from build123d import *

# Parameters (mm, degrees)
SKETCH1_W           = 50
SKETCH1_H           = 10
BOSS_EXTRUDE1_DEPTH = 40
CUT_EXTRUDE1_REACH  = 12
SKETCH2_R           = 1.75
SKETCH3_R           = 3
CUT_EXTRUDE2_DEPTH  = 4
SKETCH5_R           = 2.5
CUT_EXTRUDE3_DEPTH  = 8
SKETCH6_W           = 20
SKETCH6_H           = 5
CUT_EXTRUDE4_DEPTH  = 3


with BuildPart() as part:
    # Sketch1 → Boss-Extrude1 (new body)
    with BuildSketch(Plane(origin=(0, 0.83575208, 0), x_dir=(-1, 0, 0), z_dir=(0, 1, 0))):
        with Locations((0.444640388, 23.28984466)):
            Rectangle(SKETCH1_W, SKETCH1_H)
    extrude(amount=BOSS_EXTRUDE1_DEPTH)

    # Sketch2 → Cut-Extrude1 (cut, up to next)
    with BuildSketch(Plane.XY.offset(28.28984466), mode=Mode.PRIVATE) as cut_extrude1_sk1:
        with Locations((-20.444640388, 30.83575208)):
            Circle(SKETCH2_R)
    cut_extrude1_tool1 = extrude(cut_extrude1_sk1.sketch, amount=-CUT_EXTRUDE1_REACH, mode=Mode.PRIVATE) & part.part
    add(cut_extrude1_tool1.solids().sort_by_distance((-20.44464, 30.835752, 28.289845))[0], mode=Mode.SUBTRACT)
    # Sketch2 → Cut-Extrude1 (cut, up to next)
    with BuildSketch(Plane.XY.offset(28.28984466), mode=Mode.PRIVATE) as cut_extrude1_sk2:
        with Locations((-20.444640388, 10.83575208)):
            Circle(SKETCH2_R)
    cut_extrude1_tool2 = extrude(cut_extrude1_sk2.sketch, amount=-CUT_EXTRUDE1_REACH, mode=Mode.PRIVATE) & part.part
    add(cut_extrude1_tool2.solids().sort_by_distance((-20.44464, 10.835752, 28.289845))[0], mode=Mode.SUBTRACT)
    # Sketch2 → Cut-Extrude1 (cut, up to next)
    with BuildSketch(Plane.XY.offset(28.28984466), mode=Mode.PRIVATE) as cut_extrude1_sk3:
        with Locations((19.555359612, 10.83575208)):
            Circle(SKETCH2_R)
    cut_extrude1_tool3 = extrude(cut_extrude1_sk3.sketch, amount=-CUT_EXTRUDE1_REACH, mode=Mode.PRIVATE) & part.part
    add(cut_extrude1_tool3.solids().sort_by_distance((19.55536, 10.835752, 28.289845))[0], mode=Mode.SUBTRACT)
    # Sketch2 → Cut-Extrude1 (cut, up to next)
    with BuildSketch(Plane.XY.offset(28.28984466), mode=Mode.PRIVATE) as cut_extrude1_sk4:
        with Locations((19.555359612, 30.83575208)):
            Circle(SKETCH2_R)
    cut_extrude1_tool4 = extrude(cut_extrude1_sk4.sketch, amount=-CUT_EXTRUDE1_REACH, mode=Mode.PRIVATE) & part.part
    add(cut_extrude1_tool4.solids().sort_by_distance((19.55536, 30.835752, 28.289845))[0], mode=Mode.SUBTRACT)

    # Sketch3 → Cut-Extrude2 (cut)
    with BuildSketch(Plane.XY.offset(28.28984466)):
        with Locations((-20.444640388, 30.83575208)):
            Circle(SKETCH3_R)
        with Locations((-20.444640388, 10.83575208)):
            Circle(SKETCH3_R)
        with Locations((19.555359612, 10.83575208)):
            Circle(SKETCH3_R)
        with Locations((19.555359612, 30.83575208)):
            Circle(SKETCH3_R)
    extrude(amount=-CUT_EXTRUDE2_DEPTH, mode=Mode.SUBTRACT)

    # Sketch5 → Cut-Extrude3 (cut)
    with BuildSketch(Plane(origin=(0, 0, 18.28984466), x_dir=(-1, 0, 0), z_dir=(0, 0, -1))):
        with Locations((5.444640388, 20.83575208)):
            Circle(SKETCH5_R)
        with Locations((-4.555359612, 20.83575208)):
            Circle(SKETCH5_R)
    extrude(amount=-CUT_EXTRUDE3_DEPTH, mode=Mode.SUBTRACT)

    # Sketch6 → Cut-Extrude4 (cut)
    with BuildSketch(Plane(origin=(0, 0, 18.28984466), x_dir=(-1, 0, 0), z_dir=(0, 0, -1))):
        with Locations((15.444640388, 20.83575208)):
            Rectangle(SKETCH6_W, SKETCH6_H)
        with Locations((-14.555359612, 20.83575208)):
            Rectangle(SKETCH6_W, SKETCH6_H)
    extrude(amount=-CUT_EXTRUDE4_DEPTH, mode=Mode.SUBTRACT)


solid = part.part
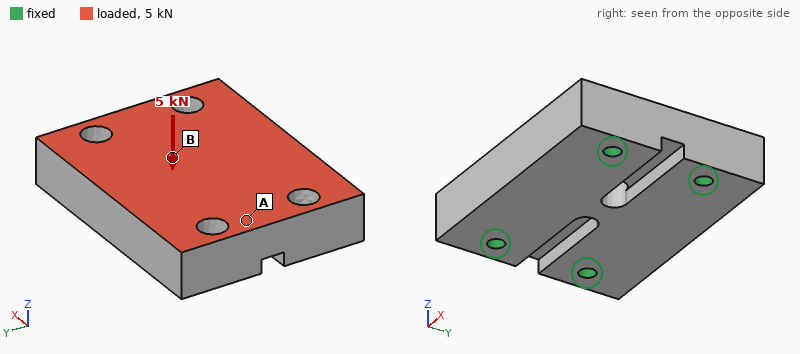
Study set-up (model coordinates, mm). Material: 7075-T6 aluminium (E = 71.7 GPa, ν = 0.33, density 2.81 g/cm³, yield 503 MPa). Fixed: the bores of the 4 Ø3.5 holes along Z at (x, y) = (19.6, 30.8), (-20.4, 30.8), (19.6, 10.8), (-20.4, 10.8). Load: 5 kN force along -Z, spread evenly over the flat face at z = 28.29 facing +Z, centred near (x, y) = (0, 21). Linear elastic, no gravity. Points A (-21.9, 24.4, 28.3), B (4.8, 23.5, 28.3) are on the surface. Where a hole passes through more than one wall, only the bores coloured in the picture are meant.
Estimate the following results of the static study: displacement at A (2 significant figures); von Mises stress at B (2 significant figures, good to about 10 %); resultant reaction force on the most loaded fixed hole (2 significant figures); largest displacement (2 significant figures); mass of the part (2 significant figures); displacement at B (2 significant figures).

2.5 µm
16 MPa
1.3 kN
11 µm
52 g
8.5 µm
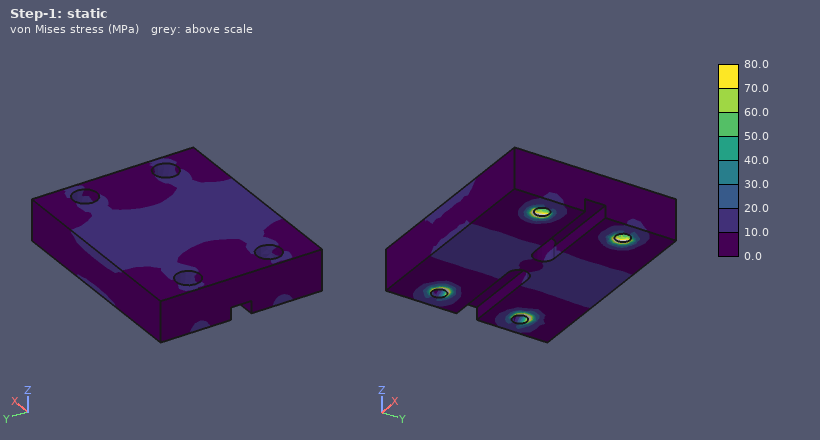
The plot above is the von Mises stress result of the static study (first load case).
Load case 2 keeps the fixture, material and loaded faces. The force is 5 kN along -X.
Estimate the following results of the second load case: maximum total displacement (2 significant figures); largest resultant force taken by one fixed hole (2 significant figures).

3.8 µm
1.3 kN
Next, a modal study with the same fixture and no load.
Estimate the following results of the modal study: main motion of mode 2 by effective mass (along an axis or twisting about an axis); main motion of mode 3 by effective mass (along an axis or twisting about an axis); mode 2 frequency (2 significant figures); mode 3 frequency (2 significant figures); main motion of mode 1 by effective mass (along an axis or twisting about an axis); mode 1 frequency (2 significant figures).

twisting about X
along Y
19 kHz
28 kHz
along Z
17 kHz
